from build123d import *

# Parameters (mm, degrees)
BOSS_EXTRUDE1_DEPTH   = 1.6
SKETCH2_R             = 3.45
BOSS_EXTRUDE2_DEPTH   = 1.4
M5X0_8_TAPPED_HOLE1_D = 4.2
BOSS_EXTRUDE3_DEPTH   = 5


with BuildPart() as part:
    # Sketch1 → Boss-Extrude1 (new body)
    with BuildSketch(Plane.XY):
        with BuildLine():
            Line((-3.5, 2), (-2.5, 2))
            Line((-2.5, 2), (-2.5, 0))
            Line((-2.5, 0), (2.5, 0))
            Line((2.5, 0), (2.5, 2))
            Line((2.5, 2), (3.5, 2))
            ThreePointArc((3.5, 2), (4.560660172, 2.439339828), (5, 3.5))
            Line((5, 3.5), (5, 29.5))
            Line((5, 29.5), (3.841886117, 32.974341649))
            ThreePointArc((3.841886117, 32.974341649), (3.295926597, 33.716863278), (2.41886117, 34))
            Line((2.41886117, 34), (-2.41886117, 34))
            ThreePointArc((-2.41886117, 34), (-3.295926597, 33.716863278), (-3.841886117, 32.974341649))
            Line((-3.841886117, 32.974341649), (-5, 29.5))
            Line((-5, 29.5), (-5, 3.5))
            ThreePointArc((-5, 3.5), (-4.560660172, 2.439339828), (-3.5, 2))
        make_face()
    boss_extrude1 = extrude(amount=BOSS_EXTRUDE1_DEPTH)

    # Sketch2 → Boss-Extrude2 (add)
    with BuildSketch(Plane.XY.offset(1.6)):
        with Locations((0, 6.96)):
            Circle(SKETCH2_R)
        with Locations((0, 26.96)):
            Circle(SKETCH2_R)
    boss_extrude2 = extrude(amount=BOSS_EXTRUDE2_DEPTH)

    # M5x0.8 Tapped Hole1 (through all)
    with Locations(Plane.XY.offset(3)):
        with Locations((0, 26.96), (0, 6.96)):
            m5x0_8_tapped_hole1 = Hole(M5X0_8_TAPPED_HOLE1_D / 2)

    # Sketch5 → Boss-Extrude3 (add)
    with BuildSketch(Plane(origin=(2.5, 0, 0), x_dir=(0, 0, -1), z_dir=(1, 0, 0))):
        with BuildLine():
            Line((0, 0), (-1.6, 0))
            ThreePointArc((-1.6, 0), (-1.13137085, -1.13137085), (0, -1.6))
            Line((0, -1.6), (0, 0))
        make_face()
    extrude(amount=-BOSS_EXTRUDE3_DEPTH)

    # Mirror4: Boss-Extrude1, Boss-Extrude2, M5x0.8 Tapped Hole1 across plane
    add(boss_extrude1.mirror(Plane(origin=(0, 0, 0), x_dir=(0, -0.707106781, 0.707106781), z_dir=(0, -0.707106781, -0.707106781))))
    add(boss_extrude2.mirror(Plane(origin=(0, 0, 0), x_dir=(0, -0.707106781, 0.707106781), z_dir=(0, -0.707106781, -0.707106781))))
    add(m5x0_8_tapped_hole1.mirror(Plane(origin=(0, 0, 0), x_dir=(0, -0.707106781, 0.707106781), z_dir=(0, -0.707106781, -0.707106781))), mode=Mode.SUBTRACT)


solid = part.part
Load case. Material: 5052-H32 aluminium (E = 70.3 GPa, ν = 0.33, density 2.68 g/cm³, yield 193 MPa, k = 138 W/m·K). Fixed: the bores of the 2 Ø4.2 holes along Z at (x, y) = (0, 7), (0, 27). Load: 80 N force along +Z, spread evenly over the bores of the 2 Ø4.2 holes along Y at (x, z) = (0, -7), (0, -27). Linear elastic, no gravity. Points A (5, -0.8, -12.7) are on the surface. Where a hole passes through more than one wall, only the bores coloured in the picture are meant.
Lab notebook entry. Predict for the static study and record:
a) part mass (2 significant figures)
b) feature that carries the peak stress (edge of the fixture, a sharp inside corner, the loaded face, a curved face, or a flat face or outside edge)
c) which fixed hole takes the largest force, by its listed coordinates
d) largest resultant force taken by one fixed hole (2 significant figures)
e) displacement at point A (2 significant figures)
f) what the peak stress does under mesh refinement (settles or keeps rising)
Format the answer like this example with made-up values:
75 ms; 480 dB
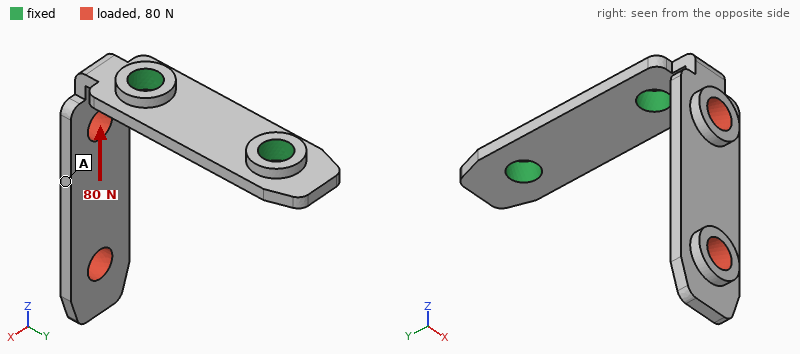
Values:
2.9 g; a sharp inside corner; (0, 7); 80 N; 0.16 mm; keeps rising
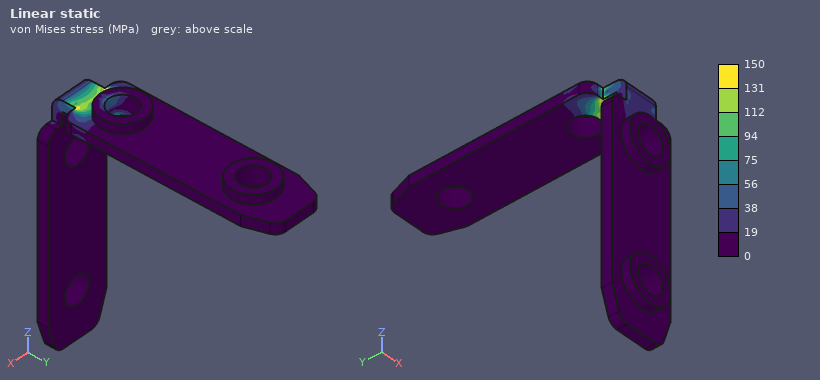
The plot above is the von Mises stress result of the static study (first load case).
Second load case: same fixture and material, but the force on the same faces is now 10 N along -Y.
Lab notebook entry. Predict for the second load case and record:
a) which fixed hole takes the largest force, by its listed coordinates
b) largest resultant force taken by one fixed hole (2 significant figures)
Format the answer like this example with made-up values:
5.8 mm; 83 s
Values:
(0, 7); 9.4 N
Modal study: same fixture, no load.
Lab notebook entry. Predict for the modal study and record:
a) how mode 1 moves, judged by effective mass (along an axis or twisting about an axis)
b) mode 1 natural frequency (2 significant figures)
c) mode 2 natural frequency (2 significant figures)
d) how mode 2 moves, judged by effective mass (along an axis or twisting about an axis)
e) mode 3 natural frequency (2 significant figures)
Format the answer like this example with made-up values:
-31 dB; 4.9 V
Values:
along Y; 730 Hz; 1300 Hz; along X; 5400 Hz
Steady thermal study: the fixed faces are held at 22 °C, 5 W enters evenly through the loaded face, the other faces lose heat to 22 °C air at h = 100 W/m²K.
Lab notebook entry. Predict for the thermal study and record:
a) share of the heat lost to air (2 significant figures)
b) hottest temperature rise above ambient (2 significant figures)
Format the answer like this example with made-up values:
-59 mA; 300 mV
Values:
47 %; 37 K
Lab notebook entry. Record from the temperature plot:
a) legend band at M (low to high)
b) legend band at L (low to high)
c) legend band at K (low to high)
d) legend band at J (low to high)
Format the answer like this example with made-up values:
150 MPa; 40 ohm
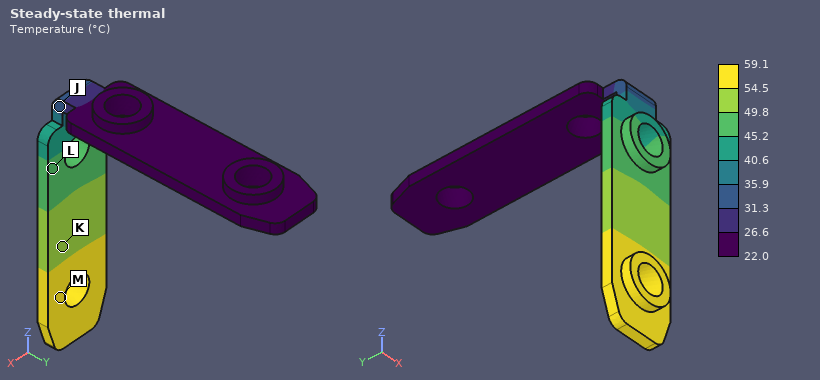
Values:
54.5 to 59.1 °C; 45.2 to 49.8 °C; 49.8 to 54.5 °C; 31.3 to 35.9 °C
